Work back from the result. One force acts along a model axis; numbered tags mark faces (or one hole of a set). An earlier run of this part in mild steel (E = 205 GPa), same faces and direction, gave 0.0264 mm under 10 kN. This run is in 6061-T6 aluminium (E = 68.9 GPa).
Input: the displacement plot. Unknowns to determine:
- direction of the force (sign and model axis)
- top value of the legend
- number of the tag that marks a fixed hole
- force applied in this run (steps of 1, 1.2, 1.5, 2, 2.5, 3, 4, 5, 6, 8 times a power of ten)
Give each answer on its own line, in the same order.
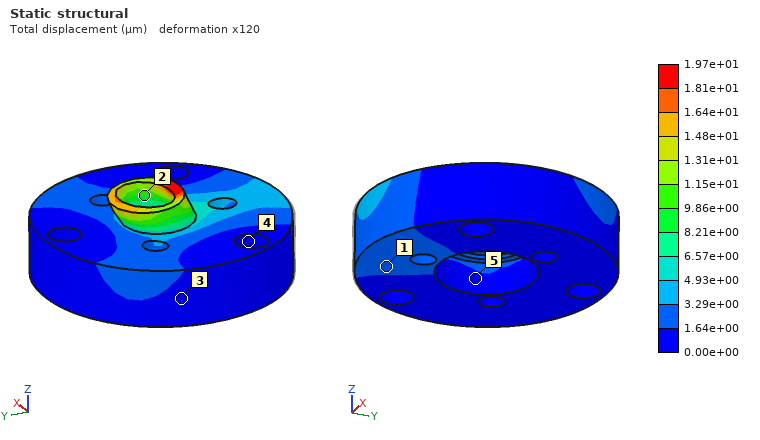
+Y
1.97e+01 µm
4
2.5 kN
